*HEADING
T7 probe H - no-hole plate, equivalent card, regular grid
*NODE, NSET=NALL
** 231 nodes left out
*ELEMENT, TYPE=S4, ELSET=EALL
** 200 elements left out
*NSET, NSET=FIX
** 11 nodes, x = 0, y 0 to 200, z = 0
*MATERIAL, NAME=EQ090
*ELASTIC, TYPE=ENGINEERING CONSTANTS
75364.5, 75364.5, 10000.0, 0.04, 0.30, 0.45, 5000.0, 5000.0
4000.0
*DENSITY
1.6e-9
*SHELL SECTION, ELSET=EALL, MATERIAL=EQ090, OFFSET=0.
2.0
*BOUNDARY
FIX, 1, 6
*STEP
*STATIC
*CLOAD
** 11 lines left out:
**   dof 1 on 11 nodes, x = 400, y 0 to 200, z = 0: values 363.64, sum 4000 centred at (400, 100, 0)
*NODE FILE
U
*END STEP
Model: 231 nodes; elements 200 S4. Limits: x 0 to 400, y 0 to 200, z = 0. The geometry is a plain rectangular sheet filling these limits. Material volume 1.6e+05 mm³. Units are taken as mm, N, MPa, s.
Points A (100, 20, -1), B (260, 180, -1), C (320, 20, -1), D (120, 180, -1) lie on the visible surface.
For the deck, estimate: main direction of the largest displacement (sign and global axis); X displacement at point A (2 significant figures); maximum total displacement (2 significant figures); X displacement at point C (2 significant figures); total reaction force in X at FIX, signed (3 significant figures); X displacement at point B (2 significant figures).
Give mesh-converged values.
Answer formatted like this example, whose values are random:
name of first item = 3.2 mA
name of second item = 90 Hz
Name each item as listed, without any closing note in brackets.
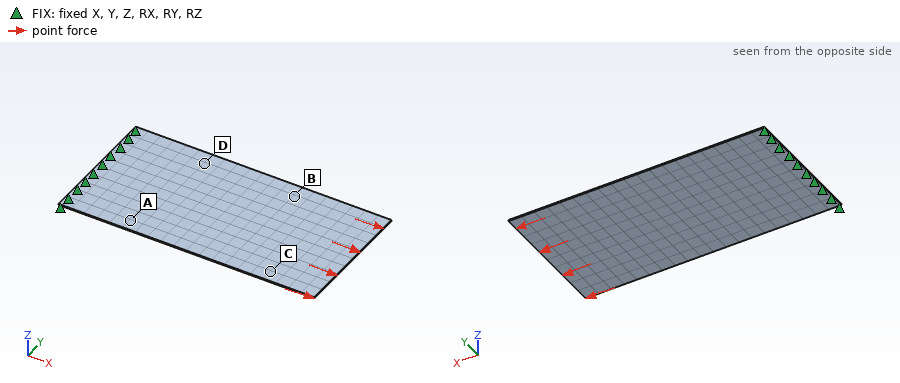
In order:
main direction of the largest displacement = +X
X displacement at point A = 0.013 mm
maximum total displacement = 0.088 mm
X displacement at point C = 0.044 mm
total reaction force in X at FIX, signed = -4000 N
X displacement at point B = 0.035 mm
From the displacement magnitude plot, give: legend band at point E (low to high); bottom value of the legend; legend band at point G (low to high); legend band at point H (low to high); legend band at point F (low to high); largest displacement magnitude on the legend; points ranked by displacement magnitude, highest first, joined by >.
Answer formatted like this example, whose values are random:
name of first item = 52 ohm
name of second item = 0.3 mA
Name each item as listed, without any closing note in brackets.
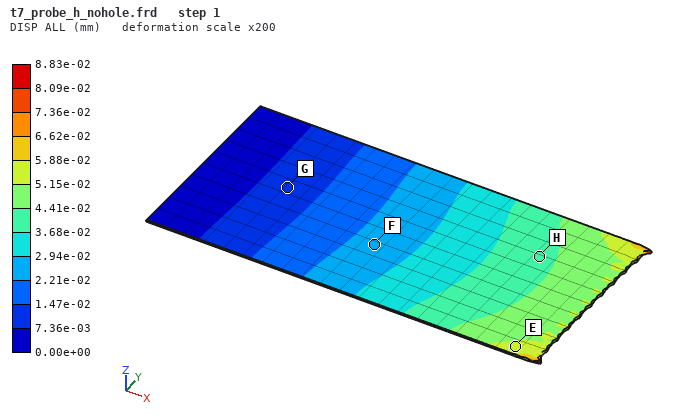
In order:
legend band at point E = 5.15e-02 to 5.88e-02 mm
bottom value of the legend = 0.00e+00 mm
legend band at point G = 7.36e-03 to 1.47e-02 mm
legend band at point H = 3.68e-02 to 4.41e-02 mm
legend band at point F = 2.21e-02 to 2.94e-02 mm
largest displacement magnitude on the legend = 8.83e-02 mm
points ranked by displacement magnitude, highest first, joined by > = E > H > F > G
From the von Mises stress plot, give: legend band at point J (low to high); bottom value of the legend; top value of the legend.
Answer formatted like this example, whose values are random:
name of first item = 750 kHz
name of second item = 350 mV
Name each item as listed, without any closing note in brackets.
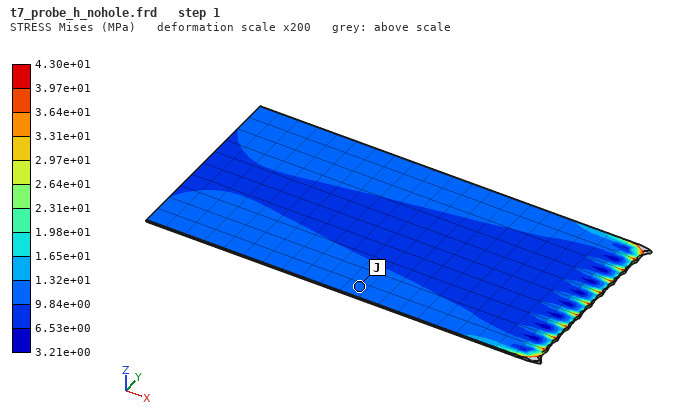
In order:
legend band at point J = 9.84e+00 to 1.32e+01 MPa
bottom value of the legend = 3.21e+00 MPa
top value of the legend = 4.30e+01 MPa
